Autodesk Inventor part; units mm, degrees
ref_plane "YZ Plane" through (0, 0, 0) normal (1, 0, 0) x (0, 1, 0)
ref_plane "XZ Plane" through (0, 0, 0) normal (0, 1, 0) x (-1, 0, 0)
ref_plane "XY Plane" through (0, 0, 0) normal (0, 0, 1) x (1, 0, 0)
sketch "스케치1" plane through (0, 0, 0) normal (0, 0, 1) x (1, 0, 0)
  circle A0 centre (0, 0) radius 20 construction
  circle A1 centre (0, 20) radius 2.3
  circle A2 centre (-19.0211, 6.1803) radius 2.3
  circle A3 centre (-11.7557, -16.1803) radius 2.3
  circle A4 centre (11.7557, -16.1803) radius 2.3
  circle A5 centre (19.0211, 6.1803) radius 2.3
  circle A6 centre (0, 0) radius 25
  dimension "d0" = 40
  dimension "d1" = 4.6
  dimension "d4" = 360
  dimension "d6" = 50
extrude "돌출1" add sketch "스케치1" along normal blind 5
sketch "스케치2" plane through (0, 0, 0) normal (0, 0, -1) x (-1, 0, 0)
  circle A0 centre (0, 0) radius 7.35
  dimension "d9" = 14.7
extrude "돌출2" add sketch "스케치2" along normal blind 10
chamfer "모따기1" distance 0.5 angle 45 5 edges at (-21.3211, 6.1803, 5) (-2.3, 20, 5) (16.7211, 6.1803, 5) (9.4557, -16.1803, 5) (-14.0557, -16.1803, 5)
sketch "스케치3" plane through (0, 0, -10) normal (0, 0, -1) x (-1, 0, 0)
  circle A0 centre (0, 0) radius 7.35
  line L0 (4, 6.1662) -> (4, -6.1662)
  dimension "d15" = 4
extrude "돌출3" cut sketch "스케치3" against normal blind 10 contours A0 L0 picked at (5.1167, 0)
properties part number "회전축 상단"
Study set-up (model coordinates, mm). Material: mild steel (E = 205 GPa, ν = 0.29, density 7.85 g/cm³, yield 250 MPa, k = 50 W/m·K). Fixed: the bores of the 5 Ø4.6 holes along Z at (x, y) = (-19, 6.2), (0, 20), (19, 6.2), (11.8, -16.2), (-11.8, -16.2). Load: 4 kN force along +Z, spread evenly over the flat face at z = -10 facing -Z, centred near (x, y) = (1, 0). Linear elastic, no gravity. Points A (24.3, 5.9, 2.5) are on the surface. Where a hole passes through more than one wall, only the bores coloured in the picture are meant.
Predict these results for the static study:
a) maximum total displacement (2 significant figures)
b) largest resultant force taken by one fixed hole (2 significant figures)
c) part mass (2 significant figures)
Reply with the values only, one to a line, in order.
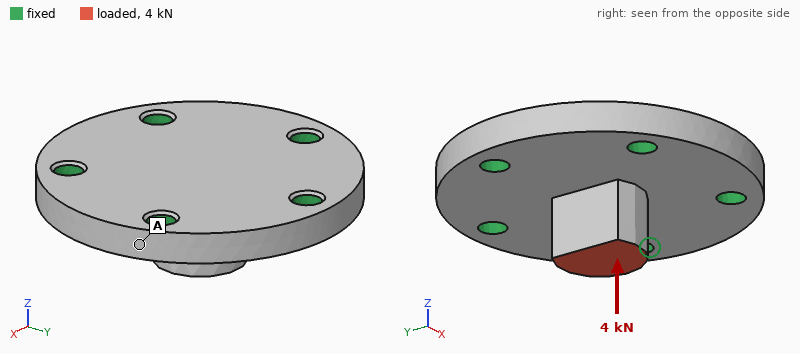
11 µm
880 N
85 g
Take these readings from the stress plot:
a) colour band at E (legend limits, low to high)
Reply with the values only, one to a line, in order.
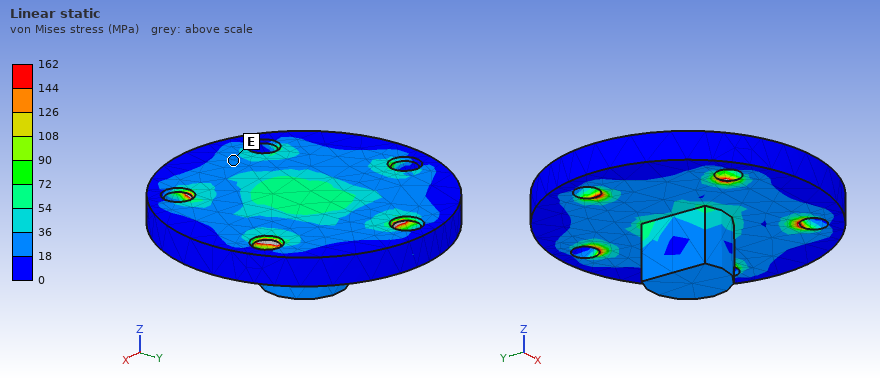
18 to 36 MPa
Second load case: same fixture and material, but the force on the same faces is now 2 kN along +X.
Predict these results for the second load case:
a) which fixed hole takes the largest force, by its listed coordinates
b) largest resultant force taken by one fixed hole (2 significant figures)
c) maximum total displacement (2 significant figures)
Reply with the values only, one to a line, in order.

(19, 6.2)
890 N
15 µm
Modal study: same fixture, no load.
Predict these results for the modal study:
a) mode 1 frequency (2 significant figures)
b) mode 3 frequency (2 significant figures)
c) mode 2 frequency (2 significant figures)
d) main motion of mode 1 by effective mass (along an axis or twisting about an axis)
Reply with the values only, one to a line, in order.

20 kHz
27 kHz
26 kHz
along Z
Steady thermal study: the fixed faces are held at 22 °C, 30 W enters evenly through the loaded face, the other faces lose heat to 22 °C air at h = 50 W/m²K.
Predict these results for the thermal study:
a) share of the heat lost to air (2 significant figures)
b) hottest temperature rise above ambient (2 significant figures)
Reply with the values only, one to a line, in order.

8.3 %
72 K
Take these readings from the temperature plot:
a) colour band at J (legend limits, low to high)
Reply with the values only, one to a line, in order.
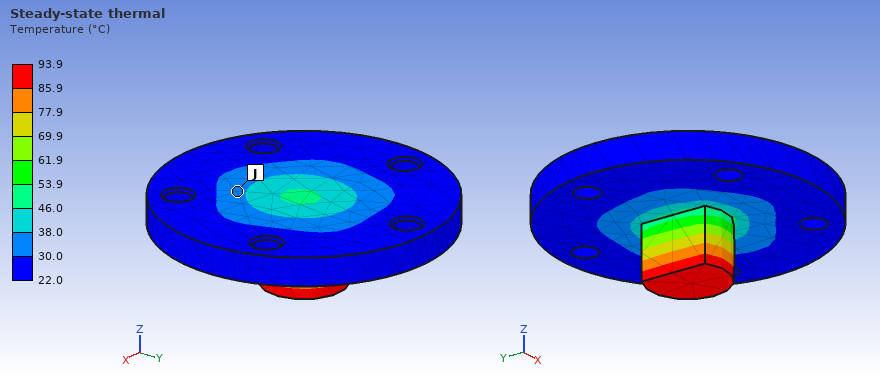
30.0 to 38.0 °C
